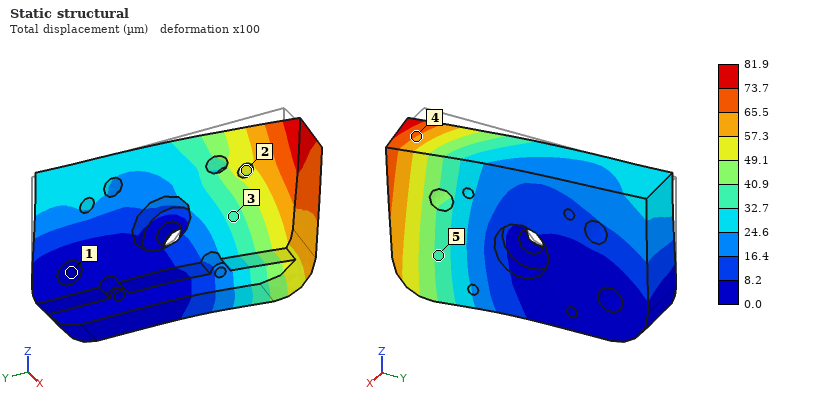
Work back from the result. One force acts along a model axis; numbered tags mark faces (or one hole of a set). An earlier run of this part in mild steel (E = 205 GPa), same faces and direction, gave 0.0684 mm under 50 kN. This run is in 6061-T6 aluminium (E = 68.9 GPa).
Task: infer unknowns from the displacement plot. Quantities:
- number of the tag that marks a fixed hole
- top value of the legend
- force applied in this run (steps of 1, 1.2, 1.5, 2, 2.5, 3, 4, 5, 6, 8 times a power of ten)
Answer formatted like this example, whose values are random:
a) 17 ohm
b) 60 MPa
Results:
a) 1
b) 81.9 µm
c) 20 kN
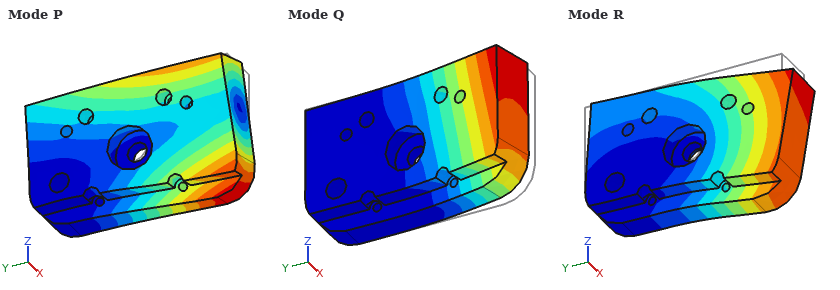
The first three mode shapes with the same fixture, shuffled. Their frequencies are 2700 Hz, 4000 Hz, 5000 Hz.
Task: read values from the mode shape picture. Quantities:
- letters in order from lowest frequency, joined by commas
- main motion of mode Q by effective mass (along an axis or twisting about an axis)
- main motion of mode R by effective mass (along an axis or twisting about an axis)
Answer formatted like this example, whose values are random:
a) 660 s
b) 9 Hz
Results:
a) Q, P, R
b) along X
c) along Z
